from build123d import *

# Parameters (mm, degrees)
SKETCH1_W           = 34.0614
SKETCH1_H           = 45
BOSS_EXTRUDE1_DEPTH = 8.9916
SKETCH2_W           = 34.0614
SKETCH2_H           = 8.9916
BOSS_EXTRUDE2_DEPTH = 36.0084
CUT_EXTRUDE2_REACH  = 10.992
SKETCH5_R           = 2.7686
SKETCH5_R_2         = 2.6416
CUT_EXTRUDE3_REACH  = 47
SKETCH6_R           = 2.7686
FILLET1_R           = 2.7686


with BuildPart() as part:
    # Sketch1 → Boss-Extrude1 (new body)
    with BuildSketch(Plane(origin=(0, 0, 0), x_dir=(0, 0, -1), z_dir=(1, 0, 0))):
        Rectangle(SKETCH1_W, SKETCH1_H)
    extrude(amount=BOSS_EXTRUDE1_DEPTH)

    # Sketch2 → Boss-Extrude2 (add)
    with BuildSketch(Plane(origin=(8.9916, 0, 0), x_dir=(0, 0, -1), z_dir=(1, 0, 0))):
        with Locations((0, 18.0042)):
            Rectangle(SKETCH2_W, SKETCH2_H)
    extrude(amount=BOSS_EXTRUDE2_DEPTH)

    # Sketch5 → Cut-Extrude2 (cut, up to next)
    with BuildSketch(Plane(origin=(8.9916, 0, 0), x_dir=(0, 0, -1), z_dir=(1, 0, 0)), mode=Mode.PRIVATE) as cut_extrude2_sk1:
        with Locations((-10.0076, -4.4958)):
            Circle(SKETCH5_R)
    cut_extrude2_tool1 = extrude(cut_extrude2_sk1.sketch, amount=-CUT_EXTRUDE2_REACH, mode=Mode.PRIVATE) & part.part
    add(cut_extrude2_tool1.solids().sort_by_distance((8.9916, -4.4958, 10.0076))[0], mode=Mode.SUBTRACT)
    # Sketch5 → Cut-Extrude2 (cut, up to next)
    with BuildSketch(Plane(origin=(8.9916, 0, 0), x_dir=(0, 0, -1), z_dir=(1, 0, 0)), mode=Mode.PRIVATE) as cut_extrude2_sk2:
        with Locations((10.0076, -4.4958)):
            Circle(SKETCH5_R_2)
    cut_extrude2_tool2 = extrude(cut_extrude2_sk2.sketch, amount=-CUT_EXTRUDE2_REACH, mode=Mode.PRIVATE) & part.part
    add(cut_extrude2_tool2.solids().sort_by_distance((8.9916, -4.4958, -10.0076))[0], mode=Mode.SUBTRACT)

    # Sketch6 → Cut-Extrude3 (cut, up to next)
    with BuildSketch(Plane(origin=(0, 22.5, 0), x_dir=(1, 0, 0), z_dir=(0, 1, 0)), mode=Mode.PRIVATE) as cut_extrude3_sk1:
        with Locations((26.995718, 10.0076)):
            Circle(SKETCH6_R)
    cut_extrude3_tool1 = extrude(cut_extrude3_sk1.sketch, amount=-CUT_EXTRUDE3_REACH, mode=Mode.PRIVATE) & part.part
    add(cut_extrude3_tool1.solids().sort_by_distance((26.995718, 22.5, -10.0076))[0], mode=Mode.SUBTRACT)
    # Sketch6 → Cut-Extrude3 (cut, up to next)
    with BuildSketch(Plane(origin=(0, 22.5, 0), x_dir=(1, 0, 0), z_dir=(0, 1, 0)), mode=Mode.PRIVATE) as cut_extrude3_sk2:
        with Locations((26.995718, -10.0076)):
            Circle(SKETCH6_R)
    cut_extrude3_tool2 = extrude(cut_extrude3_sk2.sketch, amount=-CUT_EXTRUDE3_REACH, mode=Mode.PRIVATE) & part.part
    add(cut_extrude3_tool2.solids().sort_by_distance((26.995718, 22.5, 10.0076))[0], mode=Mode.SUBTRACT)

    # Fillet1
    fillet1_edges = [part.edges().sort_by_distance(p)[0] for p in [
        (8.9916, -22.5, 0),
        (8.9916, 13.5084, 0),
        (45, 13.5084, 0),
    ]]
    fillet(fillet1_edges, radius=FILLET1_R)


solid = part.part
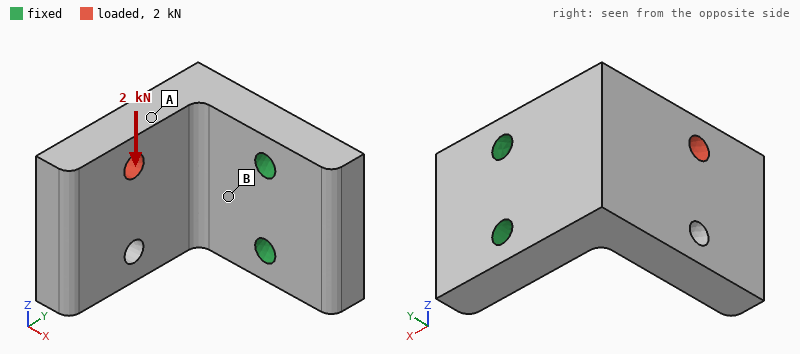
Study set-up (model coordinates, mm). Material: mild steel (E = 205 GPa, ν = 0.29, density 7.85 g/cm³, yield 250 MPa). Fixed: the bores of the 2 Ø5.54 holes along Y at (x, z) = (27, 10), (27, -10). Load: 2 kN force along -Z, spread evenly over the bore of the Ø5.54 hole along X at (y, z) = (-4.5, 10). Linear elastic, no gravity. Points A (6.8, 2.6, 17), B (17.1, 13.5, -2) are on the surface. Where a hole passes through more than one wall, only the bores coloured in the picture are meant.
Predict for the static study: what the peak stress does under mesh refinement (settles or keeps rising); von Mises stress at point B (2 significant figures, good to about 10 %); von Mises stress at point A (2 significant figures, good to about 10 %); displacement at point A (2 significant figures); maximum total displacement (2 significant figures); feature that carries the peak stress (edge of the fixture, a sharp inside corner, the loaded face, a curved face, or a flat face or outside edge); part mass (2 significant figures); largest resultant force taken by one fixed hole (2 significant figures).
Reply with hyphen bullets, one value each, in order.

- keeps rising
- 68 MPa
- 16 MPa
- 24 µm
- 44 µm
- edge of the fixture
- 190 g
- 2.7 kN
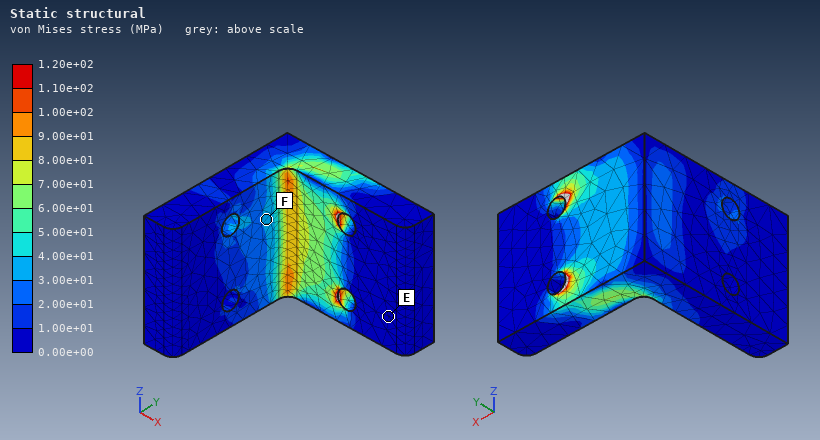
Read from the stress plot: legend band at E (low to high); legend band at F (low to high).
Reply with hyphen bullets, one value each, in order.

- 0.00e+00 to 1.00e+01 MPa
- 3.00e+01 to 4.00e+01 MPa
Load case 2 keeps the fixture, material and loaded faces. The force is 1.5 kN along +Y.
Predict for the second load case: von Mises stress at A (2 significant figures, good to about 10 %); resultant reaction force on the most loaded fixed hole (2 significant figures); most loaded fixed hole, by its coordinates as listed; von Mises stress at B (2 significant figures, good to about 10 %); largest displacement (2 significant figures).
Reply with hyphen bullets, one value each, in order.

- 15 MPa
- 1.3 kN
- (27, 10)
- 38 MPa
- 45 µm
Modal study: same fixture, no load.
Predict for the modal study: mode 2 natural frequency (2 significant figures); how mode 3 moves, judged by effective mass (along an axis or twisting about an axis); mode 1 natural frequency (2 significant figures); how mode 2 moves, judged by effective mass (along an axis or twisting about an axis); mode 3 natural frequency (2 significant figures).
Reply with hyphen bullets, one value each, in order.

- 4300 Hz
- along Y
- 2600 Hz
- along Z
- 7800 Hz
